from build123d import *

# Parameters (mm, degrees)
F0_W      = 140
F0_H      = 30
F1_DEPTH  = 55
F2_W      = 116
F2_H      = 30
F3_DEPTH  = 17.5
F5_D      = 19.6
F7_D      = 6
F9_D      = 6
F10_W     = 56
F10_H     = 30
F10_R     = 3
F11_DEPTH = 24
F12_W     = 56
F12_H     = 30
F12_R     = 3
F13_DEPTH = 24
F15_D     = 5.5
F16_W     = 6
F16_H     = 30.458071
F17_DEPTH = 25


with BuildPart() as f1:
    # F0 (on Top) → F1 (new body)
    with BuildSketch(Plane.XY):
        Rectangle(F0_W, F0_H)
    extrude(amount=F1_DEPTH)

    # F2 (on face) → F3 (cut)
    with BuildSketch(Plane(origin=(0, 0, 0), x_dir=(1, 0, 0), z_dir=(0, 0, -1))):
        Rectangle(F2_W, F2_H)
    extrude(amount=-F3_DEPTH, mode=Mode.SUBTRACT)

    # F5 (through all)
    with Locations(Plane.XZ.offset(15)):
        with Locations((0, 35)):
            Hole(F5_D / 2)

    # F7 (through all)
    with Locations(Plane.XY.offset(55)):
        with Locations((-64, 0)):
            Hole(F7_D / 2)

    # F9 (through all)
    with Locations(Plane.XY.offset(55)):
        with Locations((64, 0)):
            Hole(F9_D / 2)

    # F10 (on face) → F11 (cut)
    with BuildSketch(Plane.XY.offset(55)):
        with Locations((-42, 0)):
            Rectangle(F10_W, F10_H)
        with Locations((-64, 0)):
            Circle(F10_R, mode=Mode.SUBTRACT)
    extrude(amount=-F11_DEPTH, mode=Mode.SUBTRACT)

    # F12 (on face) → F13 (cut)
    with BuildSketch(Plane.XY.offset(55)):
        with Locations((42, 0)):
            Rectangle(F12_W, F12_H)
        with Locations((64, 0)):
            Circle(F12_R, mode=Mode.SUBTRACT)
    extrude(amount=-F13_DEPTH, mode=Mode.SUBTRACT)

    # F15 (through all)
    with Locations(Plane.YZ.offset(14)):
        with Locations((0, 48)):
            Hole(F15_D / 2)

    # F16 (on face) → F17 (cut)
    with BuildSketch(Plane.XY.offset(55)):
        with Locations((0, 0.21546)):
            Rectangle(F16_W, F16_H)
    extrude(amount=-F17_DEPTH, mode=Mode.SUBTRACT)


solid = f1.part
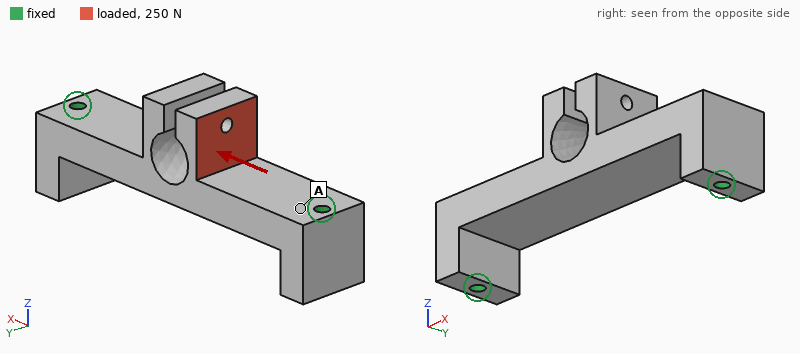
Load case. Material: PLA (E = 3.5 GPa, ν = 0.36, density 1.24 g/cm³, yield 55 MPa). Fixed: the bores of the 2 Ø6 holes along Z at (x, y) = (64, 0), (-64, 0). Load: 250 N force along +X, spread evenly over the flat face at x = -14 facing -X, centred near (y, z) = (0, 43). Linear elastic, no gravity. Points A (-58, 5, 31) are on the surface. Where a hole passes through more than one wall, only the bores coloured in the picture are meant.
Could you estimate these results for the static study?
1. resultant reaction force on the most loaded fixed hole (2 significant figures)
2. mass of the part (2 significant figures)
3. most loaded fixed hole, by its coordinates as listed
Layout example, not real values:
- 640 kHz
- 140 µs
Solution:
- 260 N
- 95 g
- (-64, 0)
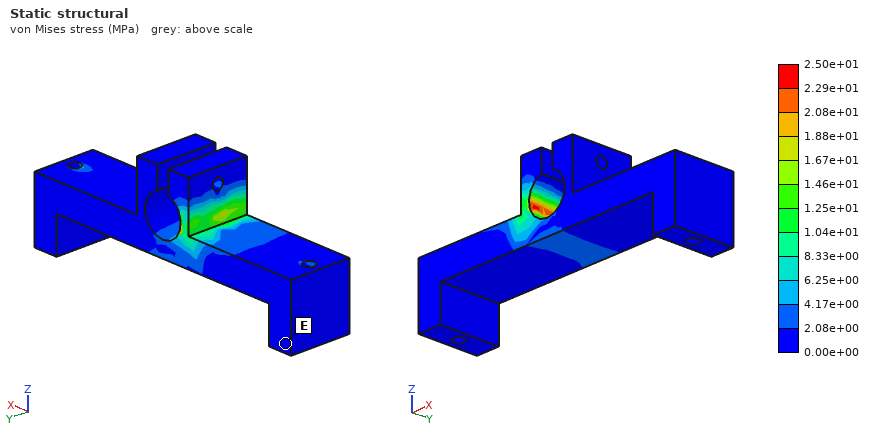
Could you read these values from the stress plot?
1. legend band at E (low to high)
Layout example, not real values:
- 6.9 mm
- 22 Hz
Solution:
- 0.00e+00 to 2.08e+00 MPa
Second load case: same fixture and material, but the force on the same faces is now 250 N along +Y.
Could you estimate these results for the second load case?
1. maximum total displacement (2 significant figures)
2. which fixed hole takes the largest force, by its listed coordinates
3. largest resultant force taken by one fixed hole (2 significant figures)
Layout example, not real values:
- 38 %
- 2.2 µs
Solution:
- 0.32 mm
- (-64, 0)
- 160 N
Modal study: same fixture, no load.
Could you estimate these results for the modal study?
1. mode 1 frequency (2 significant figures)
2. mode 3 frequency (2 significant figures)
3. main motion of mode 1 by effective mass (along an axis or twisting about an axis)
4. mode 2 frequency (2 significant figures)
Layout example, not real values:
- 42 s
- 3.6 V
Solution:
- 900 Hz
- 1300 Hz
- along Z
- 1200 Hz
